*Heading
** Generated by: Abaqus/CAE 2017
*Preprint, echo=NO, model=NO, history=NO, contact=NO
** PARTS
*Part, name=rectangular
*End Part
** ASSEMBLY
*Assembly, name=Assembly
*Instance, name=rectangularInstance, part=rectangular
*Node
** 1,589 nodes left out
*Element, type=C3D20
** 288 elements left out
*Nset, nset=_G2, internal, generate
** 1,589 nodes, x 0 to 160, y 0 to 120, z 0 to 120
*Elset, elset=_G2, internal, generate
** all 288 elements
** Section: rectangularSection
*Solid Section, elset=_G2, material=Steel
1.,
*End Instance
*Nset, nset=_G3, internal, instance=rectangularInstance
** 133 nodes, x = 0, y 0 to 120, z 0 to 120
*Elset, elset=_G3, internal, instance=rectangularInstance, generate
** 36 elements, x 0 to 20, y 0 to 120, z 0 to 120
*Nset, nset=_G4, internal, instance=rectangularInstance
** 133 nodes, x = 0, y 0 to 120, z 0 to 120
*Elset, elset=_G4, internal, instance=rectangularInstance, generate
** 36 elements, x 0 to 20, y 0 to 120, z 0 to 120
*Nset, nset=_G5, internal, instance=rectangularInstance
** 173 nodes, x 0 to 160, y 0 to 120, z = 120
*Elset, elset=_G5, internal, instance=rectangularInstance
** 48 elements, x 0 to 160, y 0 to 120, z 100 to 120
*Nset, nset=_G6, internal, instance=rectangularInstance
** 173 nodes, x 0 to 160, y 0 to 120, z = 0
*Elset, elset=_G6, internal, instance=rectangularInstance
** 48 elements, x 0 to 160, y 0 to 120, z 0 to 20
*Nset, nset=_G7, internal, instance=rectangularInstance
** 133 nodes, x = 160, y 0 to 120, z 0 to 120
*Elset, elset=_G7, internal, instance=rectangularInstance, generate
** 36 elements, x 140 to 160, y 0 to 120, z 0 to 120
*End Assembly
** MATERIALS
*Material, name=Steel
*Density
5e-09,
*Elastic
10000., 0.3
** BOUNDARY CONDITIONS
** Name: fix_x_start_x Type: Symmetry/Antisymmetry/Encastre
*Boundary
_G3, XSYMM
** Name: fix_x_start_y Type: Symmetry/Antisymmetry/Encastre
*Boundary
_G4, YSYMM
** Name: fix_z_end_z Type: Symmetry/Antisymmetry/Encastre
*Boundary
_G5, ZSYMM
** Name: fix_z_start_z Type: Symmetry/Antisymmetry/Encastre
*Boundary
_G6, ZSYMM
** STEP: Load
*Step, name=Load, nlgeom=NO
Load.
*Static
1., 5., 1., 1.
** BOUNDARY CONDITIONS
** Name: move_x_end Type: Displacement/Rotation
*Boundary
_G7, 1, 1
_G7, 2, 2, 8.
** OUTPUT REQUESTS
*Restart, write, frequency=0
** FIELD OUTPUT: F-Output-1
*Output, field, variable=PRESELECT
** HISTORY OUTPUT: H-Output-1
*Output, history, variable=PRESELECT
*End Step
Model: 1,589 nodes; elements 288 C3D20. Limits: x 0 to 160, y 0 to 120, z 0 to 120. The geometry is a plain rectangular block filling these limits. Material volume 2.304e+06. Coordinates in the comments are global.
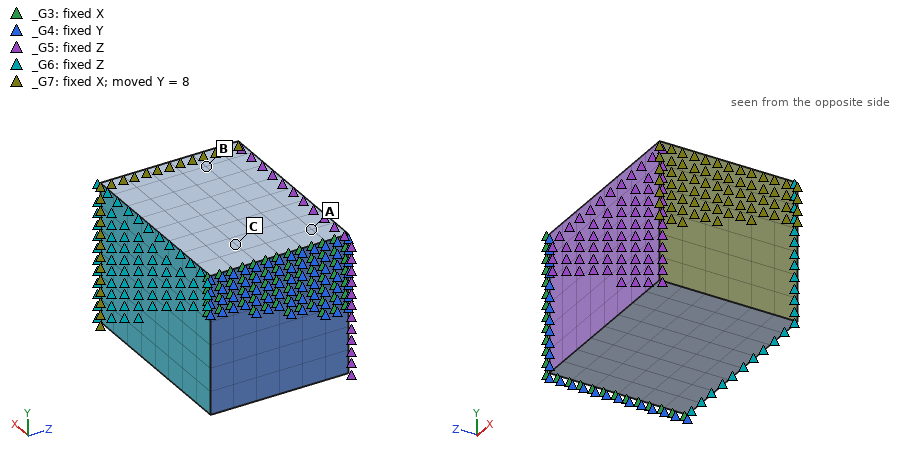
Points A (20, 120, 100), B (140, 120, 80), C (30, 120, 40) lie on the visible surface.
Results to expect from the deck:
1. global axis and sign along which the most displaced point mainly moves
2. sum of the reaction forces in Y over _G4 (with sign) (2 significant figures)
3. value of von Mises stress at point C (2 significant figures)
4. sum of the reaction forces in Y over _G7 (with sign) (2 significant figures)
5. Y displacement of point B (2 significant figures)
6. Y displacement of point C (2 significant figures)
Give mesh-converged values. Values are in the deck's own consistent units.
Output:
+Y
-1.6e+06
250
1.6e+06
7.0
1.4
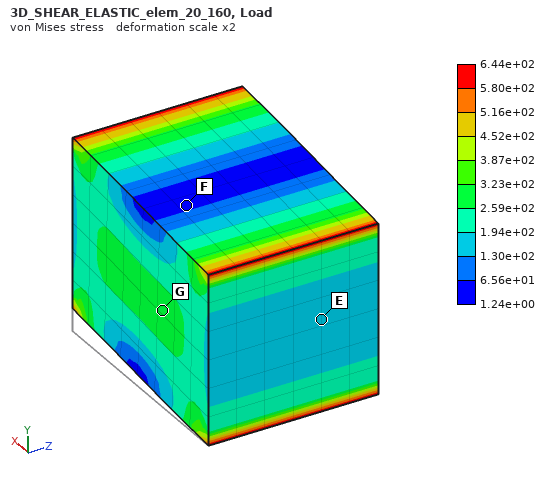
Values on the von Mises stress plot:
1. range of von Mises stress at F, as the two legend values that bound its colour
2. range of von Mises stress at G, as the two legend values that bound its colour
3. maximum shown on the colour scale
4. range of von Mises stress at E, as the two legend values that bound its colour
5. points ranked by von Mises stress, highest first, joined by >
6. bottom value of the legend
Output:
1.24e+00 to 6.56e+01
2.59e+02 to 3.23e+02
6.44e+02
1.30e+02 to 1.94e+02
G > E > F
1.24e+00
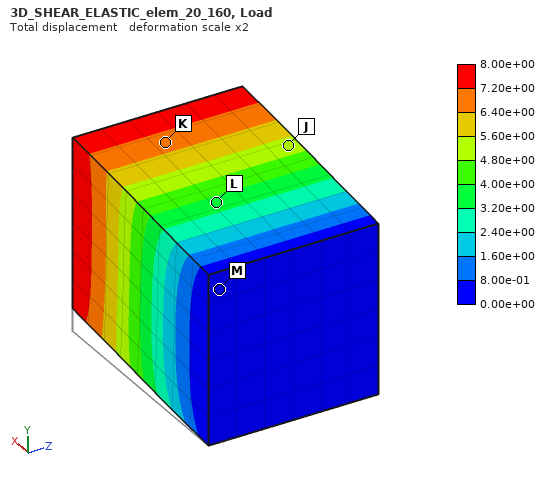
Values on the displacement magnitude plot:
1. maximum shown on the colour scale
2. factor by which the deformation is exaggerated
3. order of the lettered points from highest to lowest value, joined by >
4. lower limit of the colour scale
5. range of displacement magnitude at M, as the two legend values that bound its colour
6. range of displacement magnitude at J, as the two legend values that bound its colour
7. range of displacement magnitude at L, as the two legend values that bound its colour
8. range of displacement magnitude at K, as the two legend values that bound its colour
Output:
8.00e+00
2
K > J > L > M
0.00e+00
0.00e+00 to 8.00e-01
4.80e+00 to 5.60e+00
3.20e+00 to 4.00e+00
6.40e+00 to 7.20e+00
